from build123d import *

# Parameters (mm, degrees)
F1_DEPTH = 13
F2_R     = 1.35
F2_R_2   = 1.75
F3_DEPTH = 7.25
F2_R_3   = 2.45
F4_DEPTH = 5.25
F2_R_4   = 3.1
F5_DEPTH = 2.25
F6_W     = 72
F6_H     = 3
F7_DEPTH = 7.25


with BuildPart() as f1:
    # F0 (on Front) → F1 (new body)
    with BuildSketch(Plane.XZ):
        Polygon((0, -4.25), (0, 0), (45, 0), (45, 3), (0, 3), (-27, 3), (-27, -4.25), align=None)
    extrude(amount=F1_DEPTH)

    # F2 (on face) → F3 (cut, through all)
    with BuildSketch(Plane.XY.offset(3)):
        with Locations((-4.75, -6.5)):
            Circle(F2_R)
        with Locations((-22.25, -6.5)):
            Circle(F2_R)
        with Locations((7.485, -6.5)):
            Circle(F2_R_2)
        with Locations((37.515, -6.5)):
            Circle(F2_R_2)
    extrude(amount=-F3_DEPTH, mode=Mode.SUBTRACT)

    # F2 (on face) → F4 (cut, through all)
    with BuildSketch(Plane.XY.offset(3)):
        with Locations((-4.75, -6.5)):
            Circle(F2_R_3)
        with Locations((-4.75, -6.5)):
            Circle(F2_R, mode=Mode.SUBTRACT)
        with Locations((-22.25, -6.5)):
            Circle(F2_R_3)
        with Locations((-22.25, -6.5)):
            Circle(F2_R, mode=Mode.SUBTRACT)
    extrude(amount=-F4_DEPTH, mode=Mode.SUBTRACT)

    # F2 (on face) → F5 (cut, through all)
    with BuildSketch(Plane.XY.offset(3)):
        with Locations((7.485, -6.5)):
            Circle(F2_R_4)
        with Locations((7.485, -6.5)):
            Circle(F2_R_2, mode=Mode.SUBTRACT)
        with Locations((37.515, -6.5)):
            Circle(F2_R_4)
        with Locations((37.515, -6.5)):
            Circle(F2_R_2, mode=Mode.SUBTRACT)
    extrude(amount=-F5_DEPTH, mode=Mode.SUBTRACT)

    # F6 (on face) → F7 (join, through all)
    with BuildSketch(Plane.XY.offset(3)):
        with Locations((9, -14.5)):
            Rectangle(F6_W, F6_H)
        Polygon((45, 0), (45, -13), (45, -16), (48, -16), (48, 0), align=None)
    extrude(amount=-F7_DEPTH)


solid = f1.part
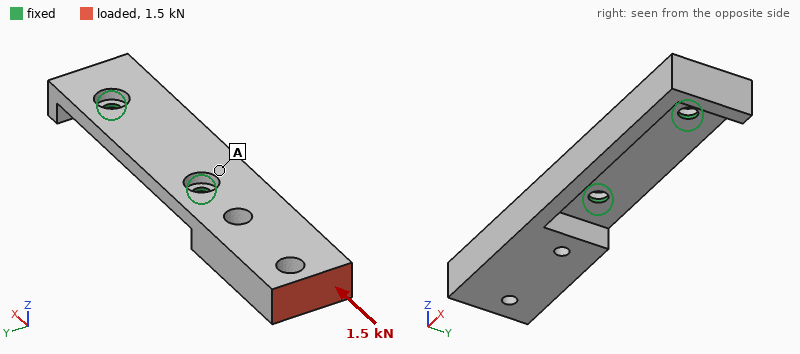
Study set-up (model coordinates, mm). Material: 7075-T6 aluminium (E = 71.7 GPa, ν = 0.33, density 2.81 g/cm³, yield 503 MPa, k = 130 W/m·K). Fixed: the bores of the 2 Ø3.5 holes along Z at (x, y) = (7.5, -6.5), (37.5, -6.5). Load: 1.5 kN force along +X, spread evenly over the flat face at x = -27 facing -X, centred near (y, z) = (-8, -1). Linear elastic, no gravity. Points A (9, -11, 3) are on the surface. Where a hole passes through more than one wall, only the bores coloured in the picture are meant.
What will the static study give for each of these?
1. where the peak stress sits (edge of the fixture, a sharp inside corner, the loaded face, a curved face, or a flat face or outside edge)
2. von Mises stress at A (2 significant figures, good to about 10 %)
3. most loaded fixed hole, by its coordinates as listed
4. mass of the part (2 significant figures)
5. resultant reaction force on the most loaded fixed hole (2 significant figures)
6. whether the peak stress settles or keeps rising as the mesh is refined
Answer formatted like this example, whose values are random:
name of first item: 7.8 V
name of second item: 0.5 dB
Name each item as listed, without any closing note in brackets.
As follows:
where the peak stress sits: edge of the fixture
von Mises stress at A: 22 MPa
most loaded fixed hole, by its coordinates as listed: (7.5, -6.5)
mass of the part: 16 g
resultant reaction force on the most loaded fixed hole: 1.2 kN
whether the peak stress settles or keeps rising as the mesh is refined: keeps rising
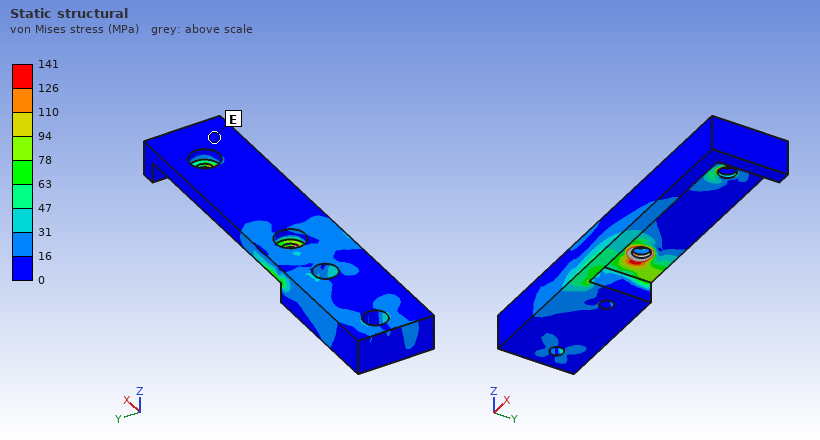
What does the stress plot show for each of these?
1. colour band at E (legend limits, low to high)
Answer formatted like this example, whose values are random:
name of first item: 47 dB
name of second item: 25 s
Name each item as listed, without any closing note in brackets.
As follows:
colour band at E: 0 to 16 MPa
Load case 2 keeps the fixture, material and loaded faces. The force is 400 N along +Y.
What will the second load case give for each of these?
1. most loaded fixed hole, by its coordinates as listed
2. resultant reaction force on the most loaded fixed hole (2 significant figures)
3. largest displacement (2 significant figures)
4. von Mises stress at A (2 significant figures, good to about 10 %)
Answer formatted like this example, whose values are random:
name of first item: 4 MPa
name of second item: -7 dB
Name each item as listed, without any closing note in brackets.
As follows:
most loaded fixed hole, by its coordinates as listed: (7.5, -6.5)
resultant reaction force on the most loaded fixed hole: 880 N
largest displacement: 0.16 mm
von Mises stress at A: 43 MPa
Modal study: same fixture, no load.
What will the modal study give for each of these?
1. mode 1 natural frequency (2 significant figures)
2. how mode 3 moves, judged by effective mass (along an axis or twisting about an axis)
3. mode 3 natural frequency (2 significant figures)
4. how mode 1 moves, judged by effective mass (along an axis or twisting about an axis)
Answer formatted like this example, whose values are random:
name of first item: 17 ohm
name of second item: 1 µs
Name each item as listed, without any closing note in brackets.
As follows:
mode 1 natural frequency: 1800 Hz
how mode 3 moves, judged by effective mass: along Y
mode 3 natural frequency: 4900 Hz
how mode 1 moves, judged by effective mass: along Z
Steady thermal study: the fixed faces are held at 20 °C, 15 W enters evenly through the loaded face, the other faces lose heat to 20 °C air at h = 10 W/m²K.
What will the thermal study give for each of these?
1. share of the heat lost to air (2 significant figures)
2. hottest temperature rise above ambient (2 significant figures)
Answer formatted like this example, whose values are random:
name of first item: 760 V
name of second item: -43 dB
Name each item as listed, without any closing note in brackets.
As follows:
share of the heat lost to air: 5.8 %
hottest temperature rise above ambient: 61 K
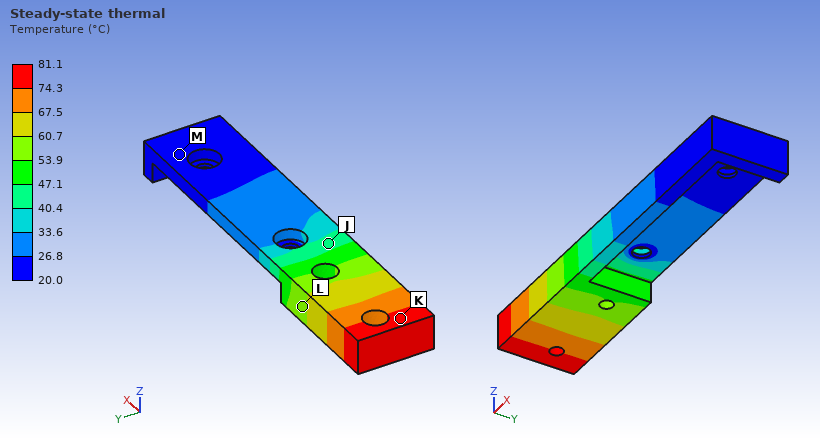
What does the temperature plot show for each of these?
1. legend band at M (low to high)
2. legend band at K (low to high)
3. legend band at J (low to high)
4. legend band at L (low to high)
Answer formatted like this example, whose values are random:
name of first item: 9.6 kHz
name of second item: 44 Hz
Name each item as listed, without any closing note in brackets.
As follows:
legend band at M: 20.0 to 26.8 °C
legend band at K: 74.3 to 81.1 °C
legend band at J: 40.4 to 47.1 °C
legend band at L: 53.9 to 60.7 °C
